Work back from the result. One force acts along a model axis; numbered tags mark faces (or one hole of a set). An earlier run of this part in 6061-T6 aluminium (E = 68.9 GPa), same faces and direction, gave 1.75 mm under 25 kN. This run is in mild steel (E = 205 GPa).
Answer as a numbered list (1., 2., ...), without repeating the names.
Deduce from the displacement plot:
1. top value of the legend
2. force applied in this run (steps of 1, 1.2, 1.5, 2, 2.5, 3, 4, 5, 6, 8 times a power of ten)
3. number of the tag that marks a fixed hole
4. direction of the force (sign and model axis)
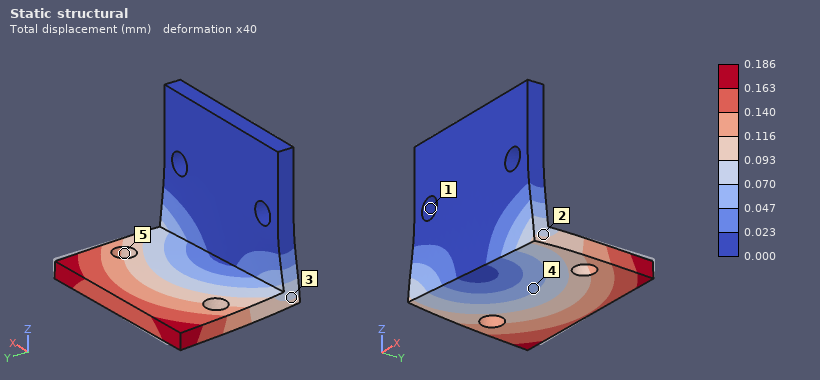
1. 0.186 mm
2. 8 kN
3. 1
4. -X
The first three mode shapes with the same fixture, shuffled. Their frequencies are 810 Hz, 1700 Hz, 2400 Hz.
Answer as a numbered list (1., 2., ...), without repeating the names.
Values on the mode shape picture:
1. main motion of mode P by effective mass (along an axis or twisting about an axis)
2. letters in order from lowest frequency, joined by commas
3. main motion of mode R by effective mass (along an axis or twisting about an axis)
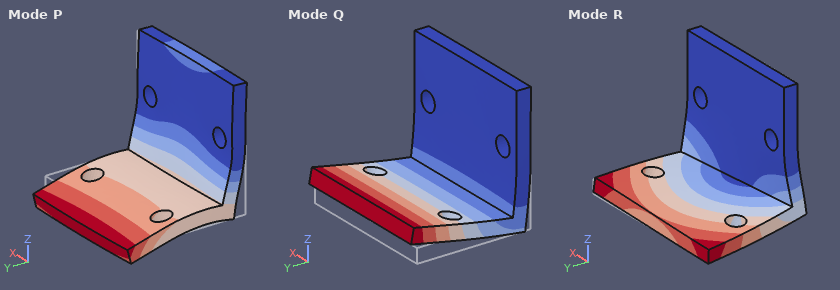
1. along Y
2. Q, R, P
3. along X
